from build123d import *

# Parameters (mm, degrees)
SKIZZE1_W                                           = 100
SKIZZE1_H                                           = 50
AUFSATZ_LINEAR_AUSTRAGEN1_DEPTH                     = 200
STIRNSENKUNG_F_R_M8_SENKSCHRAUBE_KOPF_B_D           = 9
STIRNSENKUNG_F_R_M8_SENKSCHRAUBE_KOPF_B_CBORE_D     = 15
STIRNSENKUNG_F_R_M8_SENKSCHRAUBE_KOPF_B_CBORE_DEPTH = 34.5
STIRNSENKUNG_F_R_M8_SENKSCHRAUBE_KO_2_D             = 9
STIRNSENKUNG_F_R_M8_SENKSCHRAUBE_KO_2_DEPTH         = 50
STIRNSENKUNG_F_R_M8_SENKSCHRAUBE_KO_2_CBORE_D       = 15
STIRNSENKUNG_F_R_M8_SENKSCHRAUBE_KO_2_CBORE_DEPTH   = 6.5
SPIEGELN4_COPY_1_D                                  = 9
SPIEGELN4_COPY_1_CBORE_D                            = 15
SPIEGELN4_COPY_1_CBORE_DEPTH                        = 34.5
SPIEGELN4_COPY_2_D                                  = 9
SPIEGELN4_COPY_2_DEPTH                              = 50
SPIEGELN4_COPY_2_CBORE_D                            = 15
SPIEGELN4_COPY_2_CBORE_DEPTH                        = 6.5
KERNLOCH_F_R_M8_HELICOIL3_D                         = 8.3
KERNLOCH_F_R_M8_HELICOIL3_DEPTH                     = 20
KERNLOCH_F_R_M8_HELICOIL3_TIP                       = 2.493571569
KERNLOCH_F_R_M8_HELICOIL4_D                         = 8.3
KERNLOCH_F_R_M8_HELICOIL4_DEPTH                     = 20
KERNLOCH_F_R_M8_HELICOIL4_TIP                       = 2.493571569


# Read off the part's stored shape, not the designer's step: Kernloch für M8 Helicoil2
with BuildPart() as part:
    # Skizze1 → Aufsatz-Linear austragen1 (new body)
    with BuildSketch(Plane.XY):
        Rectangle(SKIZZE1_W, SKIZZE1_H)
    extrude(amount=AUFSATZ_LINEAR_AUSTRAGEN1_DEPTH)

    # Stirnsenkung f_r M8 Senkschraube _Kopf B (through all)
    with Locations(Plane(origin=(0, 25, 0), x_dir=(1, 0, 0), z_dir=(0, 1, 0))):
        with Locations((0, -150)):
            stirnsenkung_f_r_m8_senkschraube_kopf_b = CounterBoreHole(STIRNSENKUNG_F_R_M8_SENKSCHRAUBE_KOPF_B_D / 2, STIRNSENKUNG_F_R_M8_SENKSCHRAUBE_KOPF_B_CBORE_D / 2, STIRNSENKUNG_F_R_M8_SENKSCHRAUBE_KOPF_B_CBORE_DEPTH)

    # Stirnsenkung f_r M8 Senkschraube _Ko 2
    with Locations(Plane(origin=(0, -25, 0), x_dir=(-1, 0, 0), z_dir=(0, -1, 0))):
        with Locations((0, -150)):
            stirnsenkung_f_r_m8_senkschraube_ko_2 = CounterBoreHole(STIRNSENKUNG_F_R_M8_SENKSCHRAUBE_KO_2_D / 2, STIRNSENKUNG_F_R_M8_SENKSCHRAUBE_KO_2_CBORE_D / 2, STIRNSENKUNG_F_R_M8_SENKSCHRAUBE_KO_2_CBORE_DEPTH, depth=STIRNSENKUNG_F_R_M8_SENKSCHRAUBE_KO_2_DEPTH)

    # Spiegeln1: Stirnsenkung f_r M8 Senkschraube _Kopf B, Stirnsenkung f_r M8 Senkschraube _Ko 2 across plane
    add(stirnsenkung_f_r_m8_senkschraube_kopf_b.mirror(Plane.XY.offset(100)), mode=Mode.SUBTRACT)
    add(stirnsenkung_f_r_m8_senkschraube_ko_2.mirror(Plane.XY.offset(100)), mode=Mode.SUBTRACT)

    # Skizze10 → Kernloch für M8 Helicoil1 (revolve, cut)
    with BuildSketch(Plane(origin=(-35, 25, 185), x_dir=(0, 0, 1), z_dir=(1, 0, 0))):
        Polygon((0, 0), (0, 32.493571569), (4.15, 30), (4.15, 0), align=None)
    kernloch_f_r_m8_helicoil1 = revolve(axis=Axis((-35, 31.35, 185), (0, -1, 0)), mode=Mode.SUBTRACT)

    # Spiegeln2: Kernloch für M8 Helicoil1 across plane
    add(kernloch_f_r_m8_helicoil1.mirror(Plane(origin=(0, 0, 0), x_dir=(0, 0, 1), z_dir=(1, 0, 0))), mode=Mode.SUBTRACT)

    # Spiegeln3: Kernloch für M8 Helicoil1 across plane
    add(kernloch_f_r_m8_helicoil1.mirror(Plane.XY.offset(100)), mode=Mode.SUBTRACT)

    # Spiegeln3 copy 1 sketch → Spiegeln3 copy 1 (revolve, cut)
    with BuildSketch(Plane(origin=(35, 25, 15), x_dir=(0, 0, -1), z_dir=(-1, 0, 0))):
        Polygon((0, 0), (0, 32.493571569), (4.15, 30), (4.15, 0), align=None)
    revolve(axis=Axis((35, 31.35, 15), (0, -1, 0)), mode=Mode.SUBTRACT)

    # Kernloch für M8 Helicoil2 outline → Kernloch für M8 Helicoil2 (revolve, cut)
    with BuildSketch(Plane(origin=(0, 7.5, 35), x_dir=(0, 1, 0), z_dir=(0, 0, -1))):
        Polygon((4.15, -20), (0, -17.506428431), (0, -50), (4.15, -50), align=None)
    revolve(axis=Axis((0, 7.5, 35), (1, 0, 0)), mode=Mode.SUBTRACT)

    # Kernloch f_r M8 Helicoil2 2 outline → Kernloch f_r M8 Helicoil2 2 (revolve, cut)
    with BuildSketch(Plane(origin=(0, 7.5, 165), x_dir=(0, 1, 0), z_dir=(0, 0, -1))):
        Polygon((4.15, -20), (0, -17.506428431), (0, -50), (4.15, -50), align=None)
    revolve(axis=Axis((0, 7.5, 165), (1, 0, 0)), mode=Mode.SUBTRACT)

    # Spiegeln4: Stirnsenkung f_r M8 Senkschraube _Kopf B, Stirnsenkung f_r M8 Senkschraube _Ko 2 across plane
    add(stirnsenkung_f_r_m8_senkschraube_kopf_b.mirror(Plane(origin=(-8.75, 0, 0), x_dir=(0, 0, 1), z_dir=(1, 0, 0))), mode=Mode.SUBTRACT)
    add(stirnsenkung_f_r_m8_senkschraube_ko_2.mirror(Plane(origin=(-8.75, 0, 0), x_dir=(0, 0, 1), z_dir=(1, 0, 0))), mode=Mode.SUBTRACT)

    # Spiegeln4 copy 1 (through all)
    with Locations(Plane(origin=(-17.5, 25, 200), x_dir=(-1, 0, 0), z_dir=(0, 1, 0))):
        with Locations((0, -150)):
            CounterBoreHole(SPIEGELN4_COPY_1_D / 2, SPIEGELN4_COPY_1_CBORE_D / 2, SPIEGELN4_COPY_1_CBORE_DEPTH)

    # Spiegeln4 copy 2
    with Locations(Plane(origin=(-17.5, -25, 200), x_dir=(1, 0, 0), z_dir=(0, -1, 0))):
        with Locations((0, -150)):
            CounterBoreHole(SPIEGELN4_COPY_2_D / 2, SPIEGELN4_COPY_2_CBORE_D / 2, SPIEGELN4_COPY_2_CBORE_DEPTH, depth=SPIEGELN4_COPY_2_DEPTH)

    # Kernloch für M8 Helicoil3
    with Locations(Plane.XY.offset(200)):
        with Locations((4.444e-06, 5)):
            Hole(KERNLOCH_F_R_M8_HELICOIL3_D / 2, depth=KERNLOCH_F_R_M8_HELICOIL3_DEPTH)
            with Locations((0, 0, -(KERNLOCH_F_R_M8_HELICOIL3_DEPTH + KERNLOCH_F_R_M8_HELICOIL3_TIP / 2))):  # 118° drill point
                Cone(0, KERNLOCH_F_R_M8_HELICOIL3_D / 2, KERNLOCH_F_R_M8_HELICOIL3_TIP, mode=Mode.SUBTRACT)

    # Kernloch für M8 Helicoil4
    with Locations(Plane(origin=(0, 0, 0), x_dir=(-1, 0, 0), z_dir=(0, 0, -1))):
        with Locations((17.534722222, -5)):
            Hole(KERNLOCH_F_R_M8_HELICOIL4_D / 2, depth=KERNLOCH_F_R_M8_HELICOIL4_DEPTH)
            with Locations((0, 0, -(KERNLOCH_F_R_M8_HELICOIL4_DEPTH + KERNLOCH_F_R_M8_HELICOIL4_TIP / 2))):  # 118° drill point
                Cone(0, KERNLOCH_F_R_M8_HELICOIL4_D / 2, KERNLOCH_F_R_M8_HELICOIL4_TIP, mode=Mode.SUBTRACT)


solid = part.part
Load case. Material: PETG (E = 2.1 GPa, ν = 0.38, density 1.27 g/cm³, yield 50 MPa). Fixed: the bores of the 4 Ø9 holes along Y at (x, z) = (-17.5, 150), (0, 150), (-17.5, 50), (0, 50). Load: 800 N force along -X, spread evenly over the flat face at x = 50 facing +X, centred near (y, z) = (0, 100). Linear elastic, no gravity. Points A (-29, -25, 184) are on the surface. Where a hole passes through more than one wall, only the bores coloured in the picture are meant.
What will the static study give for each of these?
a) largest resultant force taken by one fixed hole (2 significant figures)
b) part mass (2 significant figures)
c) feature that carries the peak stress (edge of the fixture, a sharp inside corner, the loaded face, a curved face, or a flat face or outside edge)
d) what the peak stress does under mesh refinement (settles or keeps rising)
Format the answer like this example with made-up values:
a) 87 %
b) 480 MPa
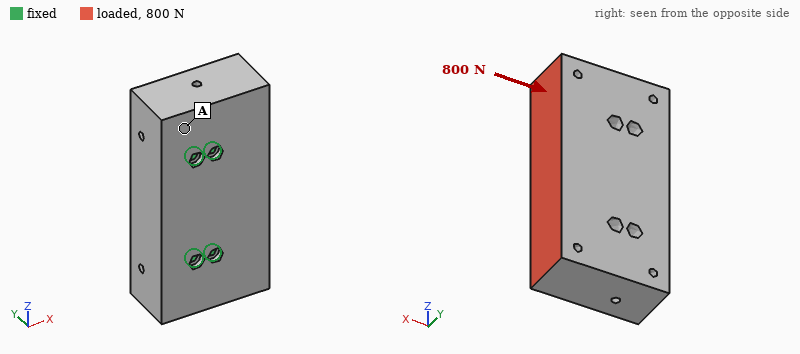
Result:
a) 300 N
b) 1.2 kg
c) edge of the fixture
d) keeps rising
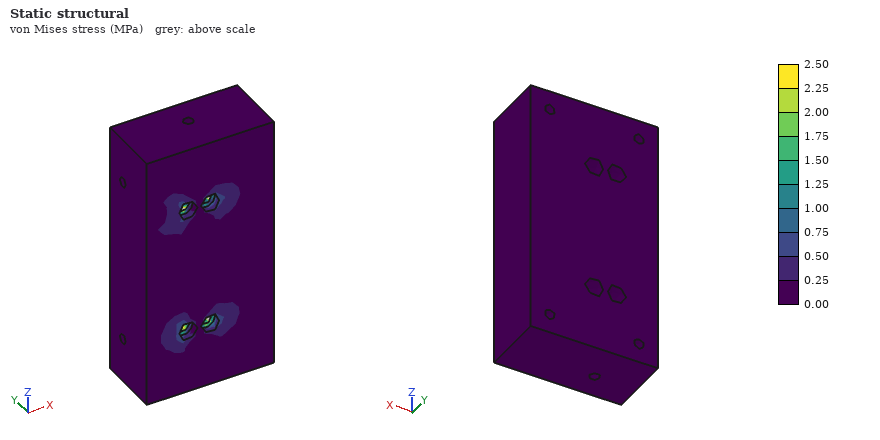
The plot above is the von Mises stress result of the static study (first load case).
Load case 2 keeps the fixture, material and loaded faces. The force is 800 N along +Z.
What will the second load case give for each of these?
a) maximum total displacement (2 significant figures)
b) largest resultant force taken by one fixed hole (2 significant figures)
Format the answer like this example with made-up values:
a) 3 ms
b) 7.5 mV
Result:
a) 34 µm
b) 400 N
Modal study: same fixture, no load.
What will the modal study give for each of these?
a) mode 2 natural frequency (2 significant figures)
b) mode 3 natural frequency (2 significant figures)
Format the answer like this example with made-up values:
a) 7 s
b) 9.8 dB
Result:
a) 1000 Hz
b) 1200 Hz
